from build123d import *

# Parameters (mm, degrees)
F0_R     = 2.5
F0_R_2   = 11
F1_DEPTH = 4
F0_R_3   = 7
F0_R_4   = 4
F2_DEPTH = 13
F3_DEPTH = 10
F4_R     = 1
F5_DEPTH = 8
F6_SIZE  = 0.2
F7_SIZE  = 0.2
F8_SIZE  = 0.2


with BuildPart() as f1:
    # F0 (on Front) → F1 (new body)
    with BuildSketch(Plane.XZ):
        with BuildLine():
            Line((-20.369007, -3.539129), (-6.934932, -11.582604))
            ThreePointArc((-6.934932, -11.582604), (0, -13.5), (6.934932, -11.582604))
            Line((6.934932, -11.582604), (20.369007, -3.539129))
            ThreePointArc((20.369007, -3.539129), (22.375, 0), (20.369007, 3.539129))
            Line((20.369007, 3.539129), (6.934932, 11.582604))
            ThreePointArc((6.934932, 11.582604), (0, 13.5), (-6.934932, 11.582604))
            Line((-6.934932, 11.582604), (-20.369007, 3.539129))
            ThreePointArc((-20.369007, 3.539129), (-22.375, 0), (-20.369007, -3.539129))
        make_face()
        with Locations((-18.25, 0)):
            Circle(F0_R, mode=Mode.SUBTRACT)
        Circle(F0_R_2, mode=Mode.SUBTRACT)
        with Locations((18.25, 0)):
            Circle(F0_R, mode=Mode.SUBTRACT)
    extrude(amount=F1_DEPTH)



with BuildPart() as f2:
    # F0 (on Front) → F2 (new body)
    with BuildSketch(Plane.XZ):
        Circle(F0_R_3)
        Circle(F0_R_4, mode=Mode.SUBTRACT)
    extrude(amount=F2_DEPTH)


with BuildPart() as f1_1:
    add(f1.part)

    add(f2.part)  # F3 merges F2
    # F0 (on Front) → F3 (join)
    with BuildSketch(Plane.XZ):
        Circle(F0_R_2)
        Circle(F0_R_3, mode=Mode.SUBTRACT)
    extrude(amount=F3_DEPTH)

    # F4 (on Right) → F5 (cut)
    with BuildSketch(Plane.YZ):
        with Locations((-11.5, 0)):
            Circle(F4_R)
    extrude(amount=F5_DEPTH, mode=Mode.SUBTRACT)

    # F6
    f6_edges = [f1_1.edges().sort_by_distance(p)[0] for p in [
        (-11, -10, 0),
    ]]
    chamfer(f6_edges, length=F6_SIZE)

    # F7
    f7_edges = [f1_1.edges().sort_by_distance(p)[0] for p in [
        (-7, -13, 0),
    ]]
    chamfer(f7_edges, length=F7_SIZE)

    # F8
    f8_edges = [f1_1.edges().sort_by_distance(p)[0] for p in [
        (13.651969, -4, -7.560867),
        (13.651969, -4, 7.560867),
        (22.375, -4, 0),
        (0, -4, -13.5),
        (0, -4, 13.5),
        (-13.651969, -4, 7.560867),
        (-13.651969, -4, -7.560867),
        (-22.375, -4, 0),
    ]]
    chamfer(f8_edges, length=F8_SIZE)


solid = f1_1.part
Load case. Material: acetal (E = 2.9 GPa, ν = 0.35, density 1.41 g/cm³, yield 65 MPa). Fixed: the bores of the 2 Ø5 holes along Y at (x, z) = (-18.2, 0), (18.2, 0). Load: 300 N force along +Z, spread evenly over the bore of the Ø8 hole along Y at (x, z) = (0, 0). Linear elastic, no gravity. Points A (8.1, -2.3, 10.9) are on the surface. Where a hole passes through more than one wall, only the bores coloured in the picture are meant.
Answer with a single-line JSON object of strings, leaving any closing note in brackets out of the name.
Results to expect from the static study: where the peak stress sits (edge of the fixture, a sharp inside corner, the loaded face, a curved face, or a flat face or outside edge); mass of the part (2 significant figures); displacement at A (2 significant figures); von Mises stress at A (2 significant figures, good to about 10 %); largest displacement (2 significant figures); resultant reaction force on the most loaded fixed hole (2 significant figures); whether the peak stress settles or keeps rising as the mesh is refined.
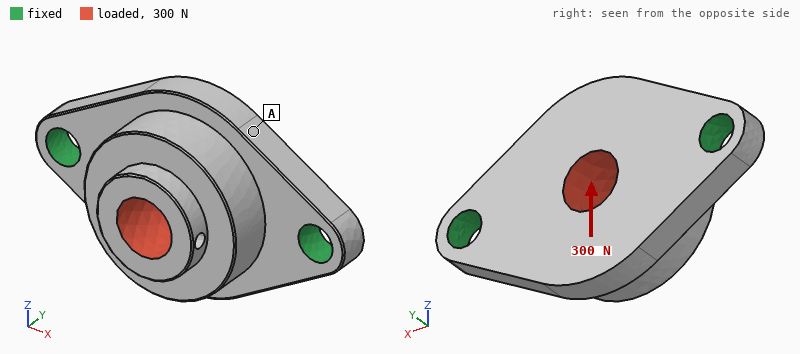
{"where the peak stress sits": "edge of the fixture", "mass of the part": "7.1 g", "displacement at A": "0.15 mm", "von Mises stress at A": "4.2 MPa", "largest displacement": "0.22 mm", "resultant reaction force on the most loaded fixed hole": "150 N", "whether the peak stress settles or keeps rising as the mesh is refined": "keeps rising"}
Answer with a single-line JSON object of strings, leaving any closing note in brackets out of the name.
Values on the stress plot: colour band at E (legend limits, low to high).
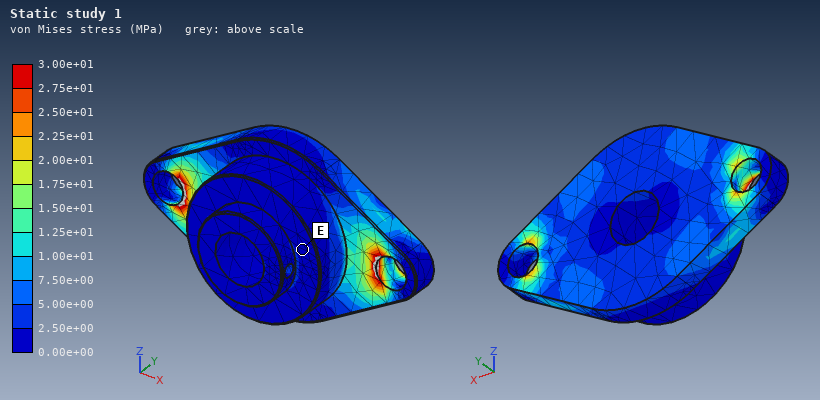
{"colour band at E": "0.00e+00 to 2.50e+00 MPa"}
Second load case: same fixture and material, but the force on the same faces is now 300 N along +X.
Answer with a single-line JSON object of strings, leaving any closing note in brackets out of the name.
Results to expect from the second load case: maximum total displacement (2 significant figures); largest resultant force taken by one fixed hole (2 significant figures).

{"maximum total displacement": "30 µm", "largest resultant force taken by one fixed hole": "160 N"}
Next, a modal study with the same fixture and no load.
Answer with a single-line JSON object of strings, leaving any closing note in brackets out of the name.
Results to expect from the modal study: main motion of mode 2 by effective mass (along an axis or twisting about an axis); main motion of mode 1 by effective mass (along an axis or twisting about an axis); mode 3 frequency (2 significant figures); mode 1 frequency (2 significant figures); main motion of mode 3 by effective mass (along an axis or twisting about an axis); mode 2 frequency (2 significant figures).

{"main motion of mode 2 by effective mass": "along Y", "main motion of mode 1 by effective mass": "along Z", "mode 3 frequency": "7100 Hz", "mode 1 frequency": "2500 Hz", "main motion of mode 3 by effective mass": "along Z", "mode 2 frequency": "4100 Hz"}
